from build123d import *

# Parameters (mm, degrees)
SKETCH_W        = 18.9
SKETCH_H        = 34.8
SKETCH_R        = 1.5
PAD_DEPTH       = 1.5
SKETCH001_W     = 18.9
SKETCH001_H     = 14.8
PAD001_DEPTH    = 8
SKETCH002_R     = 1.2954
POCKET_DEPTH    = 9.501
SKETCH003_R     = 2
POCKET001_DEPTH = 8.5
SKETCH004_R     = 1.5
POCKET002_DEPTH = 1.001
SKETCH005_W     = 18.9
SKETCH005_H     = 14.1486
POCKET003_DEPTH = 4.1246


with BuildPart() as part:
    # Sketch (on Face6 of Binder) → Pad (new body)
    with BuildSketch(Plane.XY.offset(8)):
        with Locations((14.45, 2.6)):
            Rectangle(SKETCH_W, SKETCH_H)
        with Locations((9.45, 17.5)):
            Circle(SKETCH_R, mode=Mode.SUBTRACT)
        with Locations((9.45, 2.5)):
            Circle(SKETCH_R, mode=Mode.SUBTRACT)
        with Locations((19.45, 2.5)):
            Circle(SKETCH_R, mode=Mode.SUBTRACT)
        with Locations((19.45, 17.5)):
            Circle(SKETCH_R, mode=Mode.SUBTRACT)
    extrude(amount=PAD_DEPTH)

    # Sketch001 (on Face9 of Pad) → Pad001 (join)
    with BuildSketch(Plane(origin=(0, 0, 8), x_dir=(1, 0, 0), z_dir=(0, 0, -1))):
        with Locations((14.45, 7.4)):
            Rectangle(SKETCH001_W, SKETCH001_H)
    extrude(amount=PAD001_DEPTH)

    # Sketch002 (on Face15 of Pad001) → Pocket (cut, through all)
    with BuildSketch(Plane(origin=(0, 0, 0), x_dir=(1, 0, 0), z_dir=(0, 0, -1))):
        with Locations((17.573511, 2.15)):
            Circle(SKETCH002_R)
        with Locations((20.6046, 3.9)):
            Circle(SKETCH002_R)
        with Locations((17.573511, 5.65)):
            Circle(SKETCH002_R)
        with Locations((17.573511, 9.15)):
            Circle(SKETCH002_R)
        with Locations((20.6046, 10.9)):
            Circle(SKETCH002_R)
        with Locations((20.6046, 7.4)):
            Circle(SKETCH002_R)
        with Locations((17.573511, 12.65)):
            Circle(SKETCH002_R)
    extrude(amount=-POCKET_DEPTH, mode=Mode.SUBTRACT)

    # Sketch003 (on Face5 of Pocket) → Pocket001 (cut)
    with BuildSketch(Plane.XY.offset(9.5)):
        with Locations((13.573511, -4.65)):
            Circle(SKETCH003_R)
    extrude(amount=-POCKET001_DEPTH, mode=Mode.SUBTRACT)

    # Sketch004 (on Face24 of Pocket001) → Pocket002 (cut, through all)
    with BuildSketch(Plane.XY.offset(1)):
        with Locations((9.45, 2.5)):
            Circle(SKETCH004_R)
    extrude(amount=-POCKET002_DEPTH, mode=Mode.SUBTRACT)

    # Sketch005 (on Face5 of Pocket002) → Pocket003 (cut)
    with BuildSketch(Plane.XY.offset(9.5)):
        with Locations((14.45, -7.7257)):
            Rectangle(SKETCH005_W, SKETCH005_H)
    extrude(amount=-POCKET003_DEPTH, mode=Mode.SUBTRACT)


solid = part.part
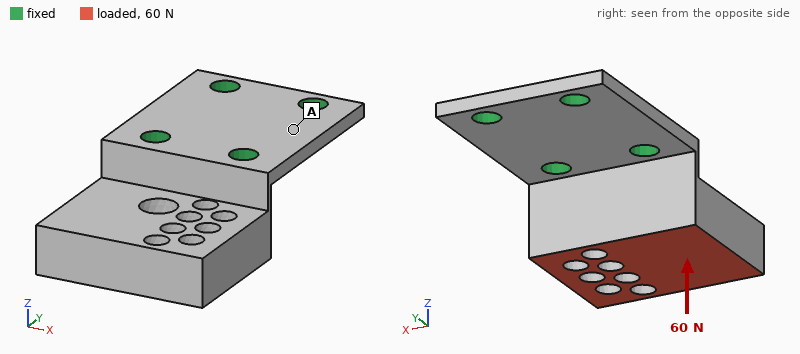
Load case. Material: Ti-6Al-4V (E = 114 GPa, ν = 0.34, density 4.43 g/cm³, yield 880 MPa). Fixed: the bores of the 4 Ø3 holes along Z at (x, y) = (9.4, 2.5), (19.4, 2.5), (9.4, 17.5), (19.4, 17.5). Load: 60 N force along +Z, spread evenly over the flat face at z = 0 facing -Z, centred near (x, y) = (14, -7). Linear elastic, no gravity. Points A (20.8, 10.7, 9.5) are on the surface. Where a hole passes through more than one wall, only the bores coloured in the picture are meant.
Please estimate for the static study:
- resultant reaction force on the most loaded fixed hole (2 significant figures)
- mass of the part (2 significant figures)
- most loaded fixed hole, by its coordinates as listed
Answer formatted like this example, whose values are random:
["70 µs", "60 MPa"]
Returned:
["34 N", "8.1 g", "(9.4, 2.5)"]
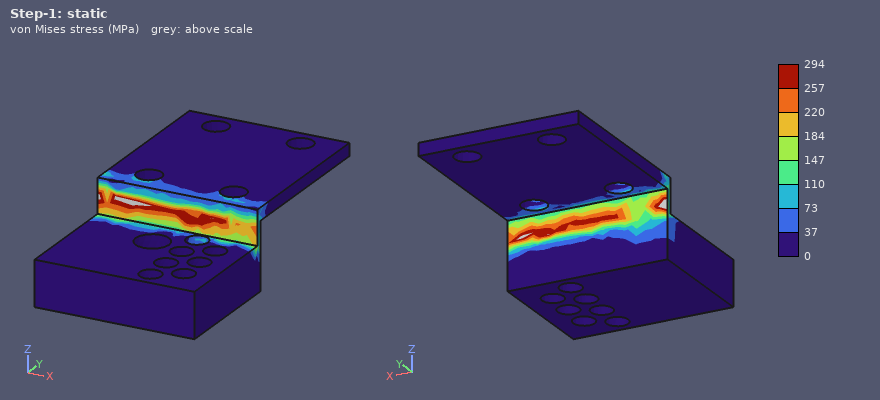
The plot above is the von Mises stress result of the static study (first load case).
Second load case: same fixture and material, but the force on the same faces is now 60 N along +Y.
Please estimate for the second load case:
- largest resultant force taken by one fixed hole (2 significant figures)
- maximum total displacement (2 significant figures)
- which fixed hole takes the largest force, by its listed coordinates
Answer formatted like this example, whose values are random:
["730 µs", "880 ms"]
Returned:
["30 N", "0.39 mm", "(9.4, 2.5)"]
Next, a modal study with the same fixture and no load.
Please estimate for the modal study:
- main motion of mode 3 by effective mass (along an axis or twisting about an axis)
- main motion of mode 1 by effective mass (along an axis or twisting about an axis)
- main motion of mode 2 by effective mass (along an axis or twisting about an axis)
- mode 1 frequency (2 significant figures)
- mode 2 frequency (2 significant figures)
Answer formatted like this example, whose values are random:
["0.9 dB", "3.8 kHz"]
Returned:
["along Y", "along Z", "along X", "920 Hz", "4700 Hz"]
